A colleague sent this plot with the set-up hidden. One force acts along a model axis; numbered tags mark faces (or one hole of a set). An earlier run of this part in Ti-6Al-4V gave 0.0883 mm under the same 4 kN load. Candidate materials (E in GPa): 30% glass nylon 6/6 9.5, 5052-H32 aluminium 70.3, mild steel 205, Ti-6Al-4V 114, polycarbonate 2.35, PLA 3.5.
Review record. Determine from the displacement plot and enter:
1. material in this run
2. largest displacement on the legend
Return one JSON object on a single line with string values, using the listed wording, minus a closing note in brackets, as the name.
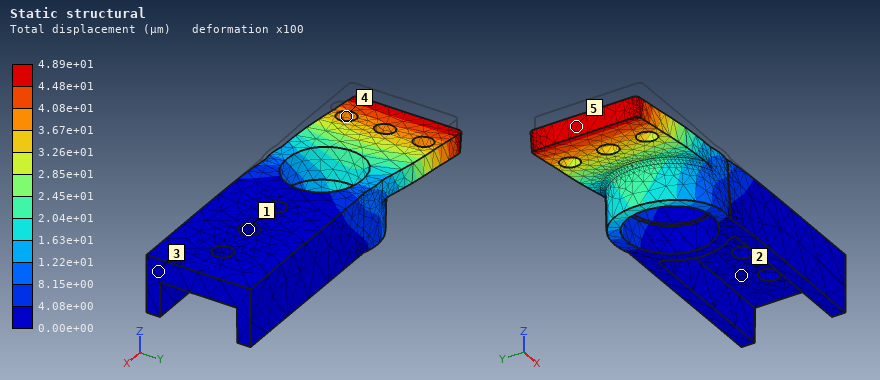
{"material in this run": "mild steel", "largest displacement on the legend": "4.89e+01 µm"}
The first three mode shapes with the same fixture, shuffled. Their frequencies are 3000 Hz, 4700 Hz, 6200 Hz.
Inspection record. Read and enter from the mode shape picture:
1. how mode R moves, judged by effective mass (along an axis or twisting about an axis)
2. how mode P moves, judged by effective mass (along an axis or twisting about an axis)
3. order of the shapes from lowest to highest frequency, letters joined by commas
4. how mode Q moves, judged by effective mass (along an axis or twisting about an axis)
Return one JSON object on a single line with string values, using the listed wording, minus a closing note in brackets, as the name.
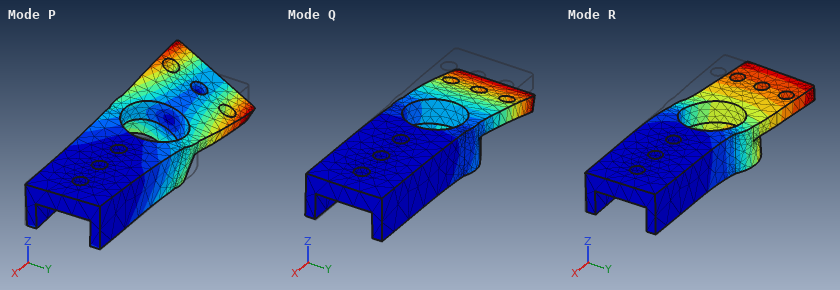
{"how mode R moves, judged by effective mass": "along Y", "how mode P moves, judged by effective mass": "twisting about X", "order of the shapes from lowest to highest frequency, letters joined by commas": "Q, R, P", "how mode Q moves, judged by effective mass": "along Z"}
